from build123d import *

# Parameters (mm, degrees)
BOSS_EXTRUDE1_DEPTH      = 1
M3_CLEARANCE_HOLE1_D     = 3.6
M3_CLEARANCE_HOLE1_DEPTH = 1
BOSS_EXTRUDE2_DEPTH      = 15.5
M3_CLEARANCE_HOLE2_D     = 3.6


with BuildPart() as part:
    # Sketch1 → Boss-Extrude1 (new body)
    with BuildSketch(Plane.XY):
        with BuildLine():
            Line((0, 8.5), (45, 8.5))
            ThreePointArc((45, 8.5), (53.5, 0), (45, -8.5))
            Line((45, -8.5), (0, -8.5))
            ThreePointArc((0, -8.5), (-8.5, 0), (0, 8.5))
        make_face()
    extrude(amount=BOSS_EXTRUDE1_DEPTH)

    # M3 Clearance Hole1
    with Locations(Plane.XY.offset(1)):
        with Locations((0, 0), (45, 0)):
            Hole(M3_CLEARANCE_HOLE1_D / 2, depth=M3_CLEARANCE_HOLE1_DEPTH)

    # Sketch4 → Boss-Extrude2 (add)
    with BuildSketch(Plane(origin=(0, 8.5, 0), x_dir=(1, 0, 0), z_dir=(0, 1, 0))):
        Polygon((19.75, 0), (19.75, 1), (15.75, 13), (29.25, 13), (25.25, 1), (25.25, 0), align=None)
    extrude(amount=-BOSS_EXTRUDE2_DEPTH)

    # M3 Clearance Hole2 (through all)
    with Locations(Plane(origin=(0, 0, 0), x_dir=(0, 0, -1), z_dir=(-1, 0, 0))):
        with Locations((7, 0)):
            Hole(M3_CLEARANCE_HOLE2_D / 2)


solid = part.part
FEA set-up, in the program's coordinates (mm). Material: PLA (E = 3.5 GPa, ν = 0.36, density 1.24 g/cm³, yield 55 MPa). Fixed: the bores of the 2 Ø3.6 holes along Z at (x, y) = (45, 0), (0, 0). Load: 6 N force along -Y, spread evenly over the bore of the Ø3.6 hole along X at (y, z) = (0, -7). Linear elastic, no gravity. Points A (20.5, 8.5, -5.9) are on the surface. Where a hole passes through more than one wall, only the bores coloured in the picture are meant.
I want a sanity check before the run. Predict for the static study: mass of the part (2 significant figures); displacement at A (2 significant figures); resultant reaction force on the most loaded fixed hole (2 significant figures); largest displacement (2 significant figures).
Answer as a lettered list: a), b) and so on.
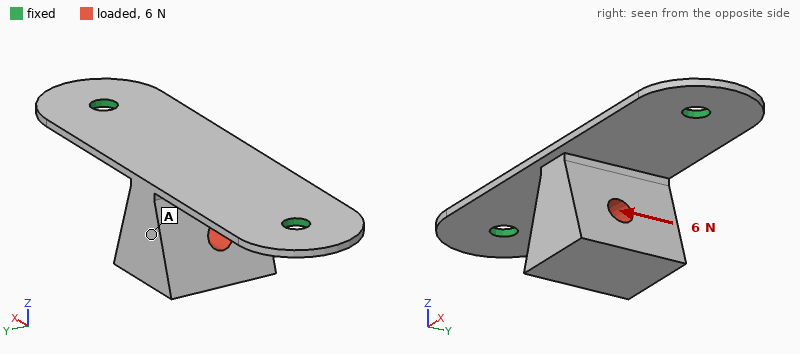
a) 3.4 g
b) 0.50 mm
c) 3.0 N
d) 0.75 mm
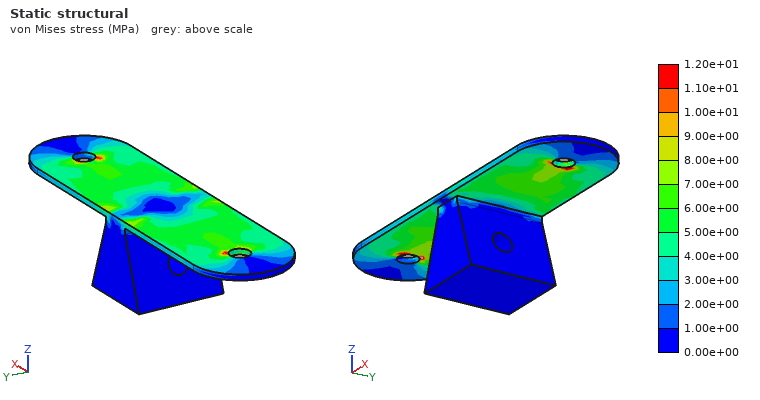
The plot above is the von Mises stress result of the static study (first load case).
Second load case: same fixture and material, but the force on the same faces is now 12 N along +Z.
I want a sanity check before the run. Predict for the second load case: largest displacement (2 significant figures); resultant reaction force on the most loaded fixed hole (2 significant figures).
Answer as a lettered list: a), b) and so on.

a) 0.72 mm
b) 6.7 N
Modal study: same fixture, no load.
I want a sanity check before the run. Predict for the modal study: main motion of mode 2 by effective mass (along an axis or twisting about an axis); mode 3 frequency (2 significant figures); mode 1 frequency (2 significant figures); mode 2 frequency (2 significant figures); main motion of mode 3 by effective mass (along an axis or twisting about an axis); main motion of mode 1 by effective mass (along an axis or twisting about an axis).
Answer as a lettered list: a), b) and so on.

a) along Z
b) 620 Hz
c) 330 Hz
d) 410 Hz
e) along X
f) along Y
